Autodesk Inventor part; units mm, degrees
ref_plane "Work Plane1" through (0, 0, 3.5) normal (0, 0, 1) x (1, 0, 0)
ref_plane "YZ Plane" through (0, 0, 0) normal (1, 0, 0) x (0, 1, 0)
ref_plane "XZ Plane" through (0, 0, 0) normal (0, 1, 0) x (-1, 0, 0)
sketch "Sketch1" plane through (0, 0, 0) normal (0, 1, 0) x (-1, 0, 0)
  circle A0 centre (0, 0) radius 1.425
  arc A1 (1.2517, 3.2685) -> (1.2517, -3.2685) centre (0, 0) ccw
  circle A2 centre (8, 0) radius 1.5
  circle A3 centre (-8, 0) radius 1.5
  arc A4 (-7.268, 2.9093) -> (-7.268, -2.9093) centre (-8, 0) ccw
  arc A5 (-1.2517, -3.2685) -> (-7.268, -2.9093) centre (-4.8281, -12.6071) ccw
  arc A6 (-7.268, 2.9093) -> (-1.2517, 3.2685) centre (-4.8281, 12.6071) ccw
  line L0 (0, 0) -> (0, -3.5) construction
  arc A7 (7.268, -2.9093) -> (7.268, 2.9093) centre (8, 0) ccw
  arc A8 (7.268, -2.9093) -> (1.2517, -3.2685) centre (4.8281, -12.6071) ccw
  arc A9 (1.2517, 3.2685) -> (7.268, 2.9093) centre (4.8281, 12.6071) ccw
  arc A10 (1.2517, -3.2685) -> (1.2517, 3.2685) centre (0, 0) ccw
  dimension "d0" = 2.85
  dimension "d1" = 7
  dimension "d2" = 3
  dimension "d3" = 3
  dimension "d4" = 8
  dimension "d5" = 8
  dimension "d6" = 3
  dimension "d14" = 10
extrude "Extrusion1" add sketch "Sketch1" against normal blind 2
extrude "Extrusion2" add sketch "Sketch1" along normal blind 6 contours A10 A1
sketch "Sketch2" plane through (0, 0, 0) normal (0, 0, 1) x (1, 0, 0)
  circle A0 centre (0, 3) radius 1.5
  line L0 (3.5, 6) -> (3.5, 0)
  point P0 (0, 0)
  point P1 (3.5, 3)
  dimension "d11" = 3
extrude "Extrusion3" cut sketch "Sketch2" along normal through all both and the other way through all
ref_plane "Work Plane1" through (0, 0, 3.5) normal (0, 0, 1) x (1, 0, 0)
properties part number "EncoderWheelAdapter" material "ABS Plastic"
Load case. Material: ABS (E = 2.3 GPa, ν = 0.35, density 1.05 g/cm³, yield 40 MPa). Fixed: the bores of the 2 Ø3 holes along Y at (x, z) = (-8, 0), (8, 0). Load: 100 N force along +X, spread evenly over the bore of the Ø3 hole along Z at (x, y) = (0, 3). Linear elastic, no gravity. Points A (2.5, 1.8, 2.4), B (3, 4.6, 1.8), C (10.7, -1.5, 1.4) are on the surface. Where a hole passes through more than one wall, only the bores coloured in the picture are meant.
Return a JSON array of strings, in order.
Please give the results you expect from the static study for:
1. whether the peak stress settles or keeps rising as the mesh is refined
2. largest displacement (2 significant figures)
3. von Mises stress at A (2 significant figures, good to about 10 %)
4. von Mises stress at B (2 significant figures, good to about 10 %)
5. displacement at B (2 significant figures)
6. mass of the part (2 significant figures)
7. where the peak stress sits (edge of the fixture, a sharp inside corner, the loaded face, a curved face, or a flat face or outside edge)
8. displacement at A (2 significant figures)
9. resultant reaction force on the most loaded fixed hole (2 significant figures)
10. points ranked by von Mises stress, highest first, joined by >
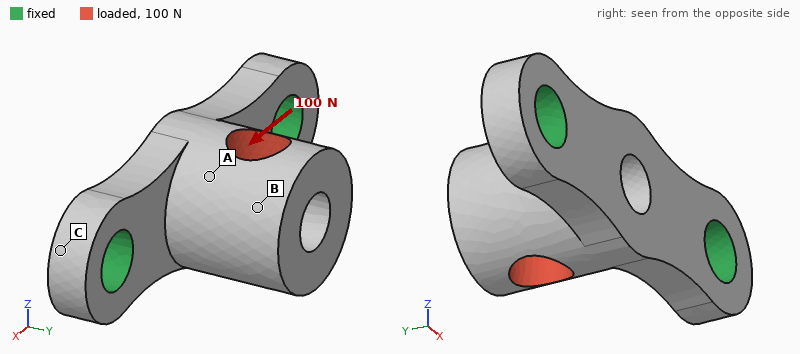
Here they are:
["keeps rising", "0.14 mm", "8.5 MPa", "4.3 MPa", "0.11 mm", "0.38 g", "edge of the fixture", "0.058 mm", "63 N", "A > B > C"]
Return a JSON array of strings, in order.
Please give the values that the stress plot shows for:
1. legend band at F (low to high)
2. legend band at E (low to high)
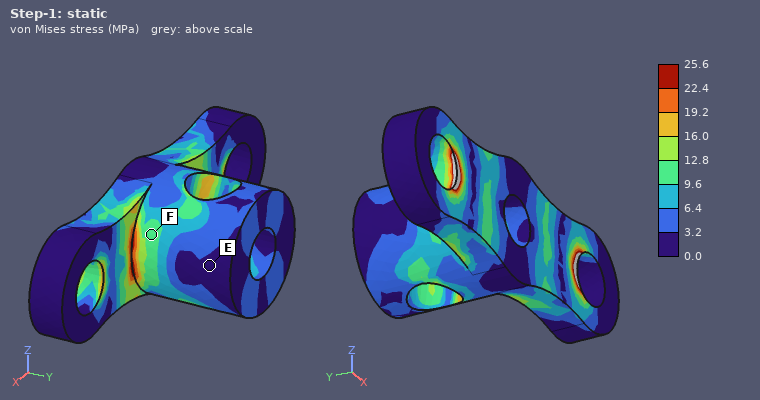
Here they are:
["9.6 to 12.8 MPa", "0.0 to 3.2 MPa"]
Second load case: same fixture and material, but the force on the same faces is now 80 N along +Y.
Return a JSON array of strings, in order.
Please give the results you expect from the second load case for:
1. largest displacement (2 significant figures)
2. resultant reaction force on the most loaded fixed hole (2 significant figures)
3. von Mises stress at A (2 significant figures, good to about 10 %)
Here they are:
["74 µm", "44 N", "3.7 MPa"]
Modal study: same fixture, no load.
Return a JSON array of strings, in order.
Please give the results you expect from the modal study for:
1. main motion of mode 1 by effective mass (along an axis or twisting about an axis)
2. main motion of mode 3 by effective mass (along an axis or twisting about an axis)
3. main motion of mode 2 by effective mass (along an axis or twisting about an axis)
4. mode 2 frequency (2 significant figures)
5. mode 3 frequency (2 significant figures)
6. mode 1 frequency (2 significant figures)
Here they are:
["along Z", "along X", "along Y", "11 kHz", "12 kHz", "5400 Hz"]
